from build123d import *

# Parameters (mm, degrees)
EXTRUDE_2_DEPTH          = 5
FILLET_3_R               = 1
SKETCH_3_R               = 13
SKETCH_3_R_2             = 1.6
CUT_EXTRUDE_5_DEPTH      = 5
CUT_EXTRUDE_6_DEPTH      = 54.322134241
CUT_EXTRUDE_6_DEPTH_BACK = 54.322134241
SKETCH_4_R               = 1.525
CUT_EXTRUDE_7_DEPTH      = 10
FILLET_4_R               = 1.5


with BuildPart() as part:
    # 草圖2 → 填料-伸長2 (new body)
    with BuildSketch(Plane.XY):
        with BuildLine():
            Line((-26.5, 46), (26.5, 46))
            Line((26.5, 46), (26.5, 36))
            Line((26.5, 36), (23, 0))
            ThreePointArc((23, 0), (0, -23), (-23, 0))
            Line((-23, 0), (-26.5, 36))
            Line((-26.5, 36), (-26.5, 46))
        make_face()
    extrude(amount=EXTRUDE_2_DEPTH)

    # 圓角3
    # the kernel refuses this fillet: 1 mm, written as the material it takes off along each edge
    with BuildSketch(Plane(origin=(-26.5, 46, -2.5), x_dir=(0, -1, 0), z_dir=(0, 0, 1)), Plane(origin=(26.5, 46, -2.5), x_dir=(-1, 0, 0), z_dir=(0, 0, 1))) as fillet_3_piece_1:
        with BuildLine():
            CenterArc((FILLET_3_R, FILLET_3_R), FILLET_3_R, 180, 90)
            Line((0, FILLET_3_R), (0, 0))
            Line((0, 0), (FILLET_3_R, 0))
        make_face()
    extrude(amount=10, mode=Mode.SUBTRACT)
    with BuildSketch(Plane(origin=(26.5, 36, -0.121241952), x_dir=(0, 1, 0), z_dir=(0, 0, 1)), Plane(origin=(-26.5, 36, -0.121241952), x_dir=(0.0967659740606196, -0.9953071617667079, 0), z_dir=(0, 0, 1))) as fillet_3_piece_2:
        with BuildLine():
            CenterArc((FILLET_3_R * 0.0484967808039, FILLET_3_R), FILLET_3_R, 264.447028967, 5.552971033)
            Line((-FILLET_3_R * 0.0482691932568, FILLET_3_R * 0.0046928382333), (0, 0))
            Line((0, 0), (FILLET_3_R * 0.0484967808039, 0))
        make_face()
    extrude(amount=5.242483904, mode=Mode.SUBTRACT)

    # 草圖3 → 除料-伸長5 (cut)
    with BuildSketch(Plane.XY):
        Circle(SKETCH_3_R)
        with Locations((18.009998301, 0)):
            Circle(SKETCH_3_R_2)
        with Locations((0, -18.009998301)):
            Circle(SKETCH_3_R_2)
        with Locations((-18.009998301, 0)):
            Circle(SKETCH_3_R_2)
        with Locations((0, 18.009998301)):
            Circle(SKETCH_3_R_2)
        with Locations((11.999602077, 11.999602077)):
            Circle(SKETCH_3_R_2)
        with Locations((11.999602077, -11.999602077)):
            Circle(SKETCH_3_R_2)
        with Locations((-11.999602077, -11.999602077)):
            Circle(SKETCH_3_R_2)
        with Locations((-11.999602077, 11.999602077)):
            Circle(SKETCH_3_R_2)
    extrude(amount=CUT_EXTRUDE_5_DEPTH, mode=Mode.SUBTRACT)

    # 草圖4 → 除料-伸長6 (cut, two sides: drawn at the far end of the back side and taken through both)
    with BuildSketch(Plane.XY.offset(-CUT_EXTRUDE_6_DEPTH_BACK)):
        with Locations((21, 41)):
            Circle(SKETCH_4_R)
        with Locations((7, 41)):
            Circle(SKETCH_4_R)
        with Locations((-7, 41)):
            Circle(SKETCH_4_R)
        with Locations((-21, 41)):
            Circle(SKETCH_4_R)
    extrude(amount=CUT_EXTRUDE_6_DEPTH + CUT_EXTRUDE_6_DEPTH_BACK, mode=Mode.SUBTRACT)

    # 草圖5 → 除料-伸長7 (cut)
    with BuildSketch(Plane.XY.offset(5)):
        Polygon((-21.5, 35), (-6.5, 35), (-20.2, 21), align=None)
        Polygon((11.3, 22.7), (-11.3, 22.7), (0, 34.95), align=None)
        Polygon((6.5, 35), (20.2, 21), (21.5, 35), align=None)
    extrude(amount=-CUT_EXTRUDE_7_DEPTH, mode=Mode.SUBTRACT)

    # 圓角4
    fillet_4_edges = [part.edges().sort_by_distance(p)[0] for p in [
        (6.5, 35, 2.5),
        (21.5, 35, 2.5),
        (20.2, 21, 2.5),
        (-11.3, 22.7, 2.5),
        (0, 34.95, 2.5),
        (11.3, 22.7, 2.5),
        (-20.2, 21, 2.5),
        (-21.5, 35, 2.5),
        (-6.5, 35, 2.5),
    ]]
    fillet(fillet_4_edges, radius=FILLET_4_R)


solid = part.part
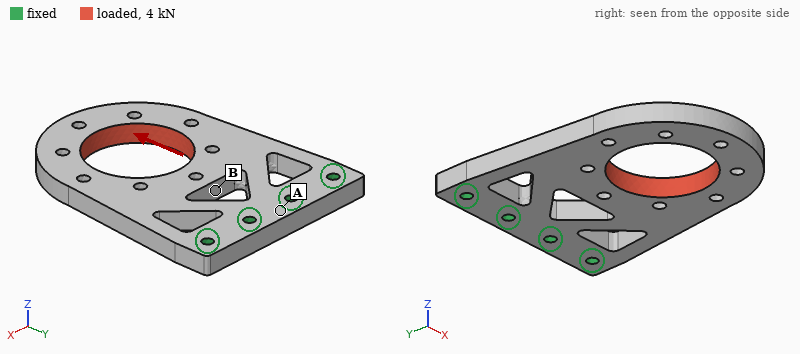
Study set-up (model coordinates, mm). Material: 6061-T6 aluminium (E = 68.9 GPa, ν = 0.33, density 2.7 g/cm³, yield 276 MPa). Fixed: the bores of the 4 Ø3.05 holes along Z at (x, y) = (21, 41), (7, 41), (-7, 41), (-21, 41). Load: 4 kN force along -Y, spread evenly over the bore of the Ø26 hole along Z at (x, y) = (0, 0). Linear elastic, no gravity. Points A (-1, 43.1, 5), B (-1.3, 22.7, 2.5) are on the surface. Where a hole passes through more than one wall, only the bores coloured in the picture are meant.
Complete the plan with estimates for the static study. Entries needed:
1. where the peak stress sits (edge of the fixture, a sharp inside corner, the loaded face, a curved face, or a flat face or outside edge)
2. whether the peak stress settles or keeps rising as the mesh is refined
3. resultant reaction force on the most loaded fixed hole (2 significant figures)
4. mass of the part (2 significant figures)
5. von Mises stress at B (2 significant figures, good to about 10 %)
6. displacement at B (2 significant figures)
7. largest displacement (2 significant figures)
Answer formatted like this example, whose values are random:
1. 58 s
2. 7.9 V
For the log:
1. a sharp inside corner
2. keeps rising
3. 1.1 kN
4. 30 g
5. 39 MPa
6. 22 µm
7. 36 µm
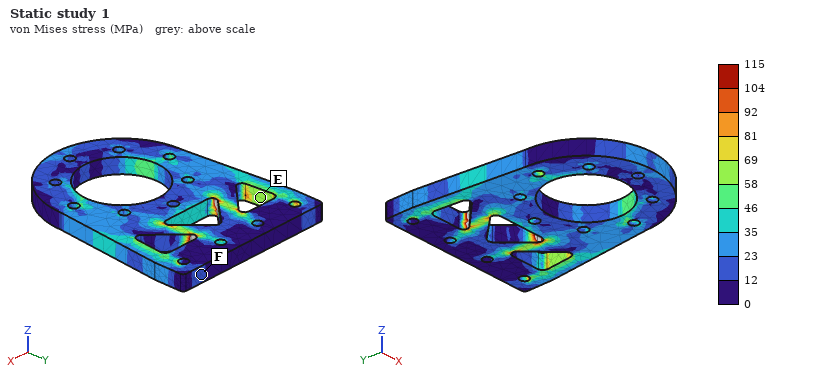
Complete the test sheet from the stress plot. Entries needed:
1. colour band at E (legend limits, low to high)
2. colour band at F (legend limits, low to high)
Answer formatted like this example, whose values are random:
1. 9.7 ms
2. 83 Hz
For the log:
1. 58 to 69 MPa
2. 12 to 23 MPa
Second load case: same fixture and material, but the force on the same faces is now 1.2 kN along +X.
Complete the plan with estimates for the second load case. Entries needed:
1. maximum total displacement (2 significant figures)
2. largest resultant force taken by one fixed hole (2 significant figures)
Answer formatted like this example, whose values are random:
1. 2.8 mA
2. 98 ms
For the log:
1. 68 µm
2. 1.1 kN
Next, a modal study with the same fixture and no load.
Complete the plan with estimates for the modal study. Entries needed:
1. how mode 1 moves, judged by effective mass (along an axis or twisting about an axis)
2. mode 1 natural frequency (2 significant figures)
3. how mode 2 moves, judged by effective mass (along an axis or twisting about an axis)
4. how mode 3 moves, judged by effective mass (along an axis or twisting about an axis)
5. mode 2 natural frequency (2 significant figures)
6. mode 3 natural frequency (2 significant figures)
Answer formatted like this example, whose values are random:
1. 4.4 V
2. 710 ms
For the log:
1. along Z
2. 990 Hz
3. twisting about Y
4. along Z
5. 3100 Hz
6. 5400 Hz
